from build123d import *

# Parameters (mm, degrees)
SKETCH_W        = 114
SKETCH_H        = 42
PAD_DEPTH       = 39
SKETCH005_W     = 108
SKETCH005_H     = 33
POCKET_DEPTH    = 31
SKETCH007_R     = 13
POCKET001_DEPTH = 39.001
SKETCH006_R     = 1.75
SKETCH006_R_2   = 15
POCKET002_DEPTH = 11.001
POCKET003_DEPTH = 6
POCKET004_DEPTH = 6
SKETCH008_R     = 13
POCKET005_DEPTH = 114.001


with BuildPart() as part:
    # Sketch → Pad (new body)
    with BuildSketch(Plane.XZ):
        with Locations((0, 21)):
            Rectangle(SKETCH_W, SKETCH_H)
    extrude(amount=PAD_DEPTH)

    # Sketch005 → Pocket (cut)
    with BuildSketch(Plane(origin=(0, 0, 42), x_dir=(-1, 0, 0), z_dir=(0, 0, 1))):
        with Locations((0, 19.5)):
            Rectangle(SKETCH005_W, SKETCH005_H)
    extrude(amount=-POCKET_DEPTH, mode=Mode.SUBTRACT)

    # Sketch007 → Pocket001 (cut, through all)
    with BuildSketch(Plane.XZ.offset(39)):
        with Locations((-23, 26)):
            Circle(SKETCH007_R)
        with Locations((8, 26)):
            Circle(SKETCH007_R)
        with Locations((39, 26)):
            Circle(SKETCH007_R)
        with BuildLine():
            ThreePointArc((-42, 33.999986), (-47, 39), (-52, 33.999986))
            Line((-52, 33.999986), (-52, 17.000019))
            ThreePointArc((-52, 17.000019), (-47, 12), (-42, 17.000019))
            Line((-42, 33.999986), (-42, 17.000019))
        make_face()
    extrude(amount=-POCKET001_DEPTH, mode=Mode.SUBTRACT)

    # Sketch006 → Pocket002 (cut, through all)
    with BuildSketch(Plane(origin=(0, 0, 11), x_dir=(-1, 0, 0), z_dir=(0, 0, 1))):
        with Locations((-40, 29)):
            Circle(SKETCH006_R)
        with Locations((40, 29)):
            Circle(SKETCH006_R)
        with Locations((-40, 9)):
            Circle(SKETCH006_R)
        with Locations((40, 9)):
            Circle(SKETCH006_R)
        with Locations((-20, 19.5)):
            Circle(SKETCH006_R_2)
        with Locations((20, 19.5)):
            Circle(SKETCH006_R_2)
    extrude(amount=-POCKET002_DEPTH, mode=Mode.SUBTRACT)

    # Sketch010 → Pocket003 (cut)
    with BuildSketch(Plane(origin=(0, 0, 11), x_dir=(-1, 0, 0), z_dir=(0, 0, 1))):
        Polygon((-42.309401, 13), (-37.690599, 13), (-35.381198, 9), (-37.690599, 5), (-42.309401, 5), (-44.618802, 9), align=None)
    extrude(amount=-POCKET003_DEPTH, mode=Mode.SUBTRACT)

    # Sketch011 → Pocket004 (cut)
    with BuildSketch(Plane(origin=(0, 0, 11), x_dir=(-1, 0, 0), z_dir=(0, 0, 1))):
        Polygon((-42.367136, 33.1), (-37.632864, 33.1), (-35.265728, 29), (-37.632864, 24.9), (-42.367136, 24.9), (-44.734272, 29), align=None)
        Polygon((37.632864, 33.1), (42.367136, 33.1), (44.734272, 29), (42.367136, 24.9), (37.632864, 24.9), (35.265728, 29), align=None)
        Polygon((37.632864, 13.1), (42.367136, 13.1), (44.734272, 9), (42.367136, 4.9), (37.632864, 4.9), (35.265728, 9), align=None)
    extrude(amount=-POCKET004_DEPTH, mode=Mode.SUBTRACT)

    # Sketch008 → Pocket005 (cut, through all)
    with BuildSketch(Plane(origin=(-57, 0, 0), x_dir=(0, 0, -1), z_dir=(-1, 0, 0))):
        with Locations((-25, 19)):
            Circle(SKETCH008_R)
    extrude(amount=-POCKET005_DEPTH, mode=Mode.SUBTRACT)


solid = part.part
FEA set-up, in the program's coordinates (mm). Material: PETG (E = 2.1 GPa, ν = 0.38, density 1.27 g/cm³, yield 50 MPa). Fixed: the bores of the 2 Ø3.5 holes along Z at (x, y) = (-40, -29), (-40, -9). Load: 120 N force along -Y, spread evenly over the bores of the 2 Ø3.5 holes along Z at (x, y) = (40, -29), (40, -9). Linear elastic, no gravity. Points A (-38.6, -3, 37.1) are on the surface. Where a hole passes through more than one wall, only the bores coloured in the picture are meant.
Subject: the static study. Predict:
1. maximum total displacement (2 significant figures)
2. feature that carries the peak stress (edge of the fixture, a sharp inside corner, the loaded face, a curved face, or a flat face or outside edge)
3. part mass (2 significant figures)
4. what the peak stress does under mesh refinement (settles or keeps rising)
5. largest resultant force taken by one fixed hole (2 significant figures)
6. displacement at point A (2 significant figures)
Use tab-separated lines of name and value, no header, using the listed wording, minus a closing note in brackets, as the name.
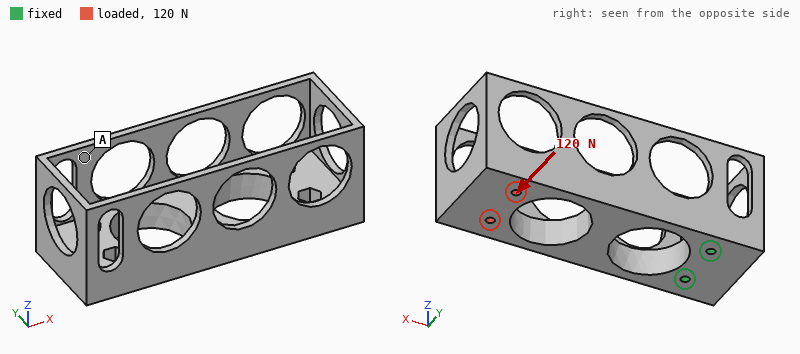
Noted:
maximum total displacement	1.2 mm
feature that carries the peak stress	edge of the fixture
part mass	57 g
what the peak stress does under mesh refinement	keeps rising
largest resultant force taken by one fixed hole	430 N
displacement at point A	0.18 mm
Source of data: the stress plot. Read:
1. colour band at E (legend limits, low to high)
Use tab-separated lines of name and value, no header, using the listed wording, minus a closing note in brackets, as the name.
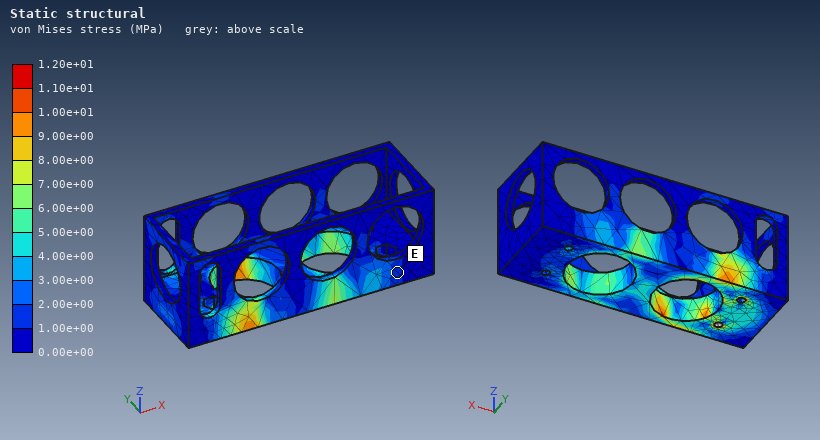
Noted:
colour band at E	1.00e+00 to 2.00e+00 MPa
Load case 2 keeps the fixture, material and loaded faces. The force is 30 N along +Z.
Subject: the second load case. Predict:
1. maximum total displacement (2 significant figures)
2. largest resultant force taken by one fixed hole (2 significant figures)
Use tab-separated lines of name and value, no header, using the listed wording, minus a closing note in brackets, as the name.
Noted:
maximum total displacement	1.4 mm
largest resultant force taken by one fixed hole	28 N
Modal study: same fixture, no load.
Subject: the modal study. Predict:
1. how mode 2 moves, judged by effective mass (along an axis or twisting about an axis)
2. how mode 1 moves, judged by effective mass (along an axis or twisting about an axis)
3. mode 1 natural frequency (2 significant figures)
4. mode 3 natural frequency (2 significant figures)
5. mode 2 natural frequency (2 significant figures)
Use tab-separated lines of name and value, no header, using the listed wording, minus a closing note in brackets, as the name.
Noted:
how mode 2 moves, judged by effective mass	along Y
how mode 1 moves, judged by effective mass	along Z
mode 1 natural frequency	160 Hz
mode 3 natural frequency	440 Hz
mode 2 natural frequency	320 Hz
